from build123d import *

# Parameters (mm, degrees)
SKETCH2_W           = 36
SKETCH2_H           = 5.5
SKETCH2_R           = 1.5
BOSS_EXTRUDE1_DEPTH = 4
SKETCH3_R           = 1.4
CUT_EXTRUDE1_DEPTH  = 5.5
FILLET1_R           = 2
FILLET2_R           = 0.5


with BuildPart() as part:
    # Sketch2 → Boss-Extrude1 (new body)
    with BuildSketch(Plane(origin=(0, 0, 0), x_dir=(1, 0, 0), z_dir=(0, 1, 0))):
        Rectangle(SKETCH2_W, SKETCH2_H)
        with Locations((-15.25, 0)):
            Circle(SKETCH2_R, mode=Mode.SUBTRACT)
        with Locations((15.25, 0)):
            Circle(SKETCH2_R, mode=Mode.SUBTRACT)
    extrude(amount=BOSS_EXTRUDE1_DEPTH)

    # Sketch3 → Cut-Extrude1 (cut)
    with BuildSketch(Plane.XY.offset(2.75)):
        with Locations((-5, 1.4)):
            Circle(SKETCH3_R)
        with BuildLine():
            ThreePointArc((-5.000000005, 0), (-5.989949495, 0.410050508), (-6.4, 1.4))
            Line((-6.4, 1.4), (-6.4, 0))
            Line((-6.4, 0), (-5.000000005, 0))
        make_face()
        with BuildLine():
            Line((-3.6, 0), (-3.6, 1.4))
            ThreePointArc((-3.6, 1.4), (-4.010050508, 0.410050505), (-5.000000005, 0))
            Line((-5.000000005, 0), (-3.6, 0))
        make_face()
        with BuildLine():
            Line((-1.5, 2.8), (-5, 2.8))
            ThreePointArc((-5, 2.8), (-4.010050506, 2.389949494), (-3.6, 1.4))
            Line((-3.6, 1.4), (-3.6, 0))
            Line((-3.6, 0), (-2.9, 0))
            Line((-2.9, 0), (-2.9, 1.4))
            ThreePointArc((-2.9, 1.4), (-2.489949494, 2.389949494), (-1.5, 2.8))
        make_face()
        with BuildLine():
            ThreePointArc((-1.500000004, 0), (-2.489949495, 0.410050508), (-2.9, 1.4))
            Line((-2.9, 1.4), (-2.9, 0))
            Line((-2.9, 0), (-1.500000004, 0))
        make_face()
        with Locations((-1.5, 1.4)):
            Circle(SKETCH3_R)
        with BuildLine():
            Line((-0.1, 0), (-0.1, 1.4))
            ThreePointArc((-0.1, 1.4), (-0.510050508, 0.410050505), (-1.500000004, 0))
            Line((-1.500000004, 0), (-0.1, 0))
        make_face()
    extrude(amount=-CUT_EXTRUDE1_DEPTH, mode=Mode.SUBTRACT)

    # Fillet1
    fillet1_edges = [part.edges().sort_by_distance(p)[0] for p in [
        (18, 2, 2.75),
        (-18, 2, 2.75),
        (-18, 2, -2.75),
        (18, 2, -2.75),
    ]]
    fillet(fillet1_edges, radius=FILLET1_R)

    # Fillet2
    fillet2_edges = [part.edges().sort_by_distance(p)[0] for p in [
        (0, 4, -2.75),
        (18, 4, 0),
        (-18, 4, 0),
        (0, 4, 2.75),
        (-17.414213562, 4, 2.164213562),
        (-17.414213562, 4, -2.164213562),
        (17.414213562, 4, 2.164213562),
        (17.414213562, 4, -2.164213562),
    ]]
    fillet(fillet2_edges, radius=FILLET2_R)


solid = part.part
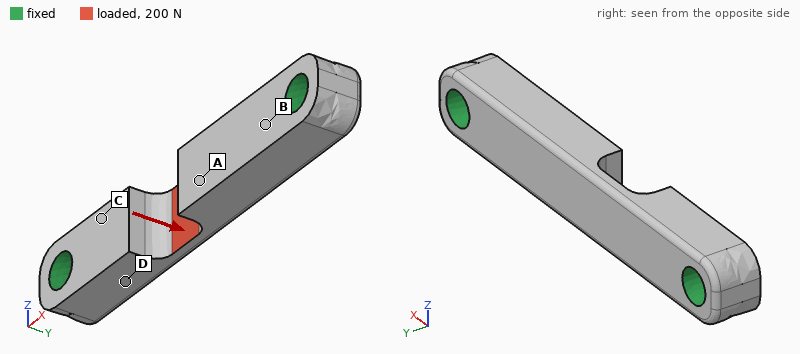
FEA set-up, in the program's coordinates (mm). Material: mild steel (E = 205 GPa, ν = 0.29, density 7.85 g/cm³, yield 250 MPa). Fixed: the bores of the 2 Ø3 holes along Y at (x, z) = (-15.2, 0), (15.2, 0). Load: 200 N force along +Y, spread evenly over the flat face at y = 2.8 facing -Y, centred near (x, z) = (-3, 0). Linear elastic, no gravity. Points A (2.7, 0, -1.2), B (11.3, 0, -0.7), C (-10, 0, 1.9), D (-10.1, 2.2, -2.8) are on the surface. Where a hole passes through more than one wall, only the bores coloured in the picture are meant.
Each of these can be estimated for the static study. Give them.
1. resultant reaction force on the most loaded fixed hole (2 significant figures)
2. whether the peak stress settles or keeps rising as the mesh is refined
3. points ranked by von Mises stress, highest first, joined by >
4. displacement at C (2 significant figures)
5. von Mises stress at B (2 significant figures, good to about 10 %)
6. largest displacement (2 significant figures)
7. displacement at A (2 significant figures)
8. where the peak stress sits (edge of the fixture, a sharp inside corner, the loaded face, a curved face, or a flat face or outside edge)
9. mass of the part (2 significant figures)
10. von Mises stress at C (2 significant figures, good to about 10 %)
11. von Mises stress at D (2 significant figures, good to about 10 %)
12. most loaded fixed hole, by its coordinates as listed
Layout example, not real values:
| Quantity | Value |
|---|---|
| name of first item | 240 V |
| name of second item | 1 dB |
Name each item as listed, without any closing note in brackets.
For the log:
| Quantity | Value |
|---|---|
| resultant reaction force on the most loaded fixed hole | 230 N |
| whether the peak stress settles or keeps rising as the mesh is refined | keeps rising |
| points ranked by von Mises stress, highest first, joined by > | B > C > D > A |
| displacement at C | 2.0 µm |
| von Mises stress at B | 48 MPa |
| largest displacement | 9.3 µm |
| displacement at A | 6.3 µm |
| where the peak stress sits | edge of the fixture |
| mass of the part | 4.9 g |
| von Mises stress at C | 37 MPa |
| von Mises stress at D | 19 MPa |
| most loaded fixed hole, by its coordinates as listed | (-15.2, 0) |
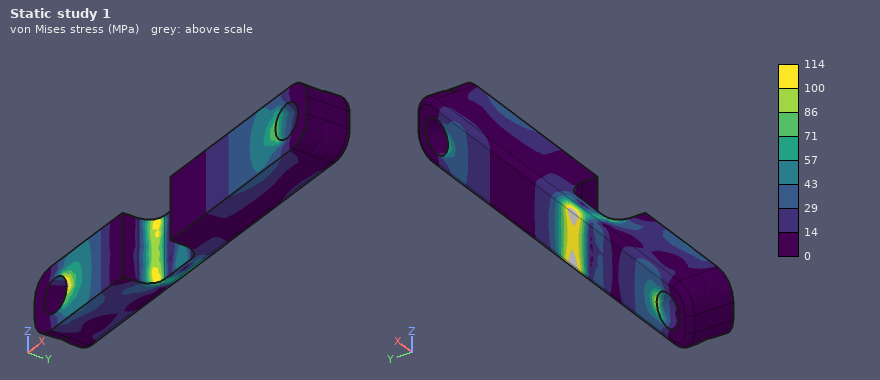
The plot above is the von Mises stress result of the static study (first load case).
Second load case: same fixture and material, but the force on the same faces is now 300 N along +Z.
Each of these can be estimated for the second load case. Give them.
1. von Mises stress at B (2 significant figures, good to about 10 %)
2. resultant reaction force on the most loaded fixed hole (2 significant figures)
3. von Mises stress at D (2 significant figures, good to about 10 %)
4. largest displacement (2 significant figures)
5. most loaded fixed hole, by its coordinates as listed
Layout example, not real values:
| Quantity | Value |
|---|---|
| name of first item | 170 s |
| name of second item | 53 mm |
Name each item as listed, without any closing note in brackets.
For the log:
| Quantity | Value |
|---|---|
| von Mises stress at B | 12 MPa |
| resultant reaction force on the most loaded fixed hole | 200 N |
| von Mises stress at D | 35 MPa |
| largest displacement | 7.9 µm |
| most loaded fixed hole, by its coordinates as listed | (-15.2, 0) |
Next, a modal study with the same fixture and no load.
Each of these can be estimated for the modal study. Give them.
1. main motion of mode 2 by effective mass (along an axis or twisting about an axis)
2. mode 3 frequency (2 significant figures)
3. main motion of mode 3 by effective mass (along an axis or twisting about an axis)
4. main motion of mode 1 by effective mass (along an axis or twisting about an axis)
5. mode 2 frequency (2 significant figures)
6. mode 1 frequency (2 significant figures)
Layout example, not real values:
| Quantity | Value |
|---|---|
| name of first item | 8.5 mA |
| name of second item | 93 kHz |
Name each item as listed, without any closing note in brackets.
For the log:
| Quantity | Value |
|---|---|
| main motion of mode 2 by effective mass | along Z |
| mode 3 frequency | 47 kHz |
| main motion of mode 3 by effective mass | twisting about X |
| main motion of mode 1 by effective mass | along Y |
| mode 2 frequency | 27 kHz |
| mode 1 frequency | 21 kHz |
